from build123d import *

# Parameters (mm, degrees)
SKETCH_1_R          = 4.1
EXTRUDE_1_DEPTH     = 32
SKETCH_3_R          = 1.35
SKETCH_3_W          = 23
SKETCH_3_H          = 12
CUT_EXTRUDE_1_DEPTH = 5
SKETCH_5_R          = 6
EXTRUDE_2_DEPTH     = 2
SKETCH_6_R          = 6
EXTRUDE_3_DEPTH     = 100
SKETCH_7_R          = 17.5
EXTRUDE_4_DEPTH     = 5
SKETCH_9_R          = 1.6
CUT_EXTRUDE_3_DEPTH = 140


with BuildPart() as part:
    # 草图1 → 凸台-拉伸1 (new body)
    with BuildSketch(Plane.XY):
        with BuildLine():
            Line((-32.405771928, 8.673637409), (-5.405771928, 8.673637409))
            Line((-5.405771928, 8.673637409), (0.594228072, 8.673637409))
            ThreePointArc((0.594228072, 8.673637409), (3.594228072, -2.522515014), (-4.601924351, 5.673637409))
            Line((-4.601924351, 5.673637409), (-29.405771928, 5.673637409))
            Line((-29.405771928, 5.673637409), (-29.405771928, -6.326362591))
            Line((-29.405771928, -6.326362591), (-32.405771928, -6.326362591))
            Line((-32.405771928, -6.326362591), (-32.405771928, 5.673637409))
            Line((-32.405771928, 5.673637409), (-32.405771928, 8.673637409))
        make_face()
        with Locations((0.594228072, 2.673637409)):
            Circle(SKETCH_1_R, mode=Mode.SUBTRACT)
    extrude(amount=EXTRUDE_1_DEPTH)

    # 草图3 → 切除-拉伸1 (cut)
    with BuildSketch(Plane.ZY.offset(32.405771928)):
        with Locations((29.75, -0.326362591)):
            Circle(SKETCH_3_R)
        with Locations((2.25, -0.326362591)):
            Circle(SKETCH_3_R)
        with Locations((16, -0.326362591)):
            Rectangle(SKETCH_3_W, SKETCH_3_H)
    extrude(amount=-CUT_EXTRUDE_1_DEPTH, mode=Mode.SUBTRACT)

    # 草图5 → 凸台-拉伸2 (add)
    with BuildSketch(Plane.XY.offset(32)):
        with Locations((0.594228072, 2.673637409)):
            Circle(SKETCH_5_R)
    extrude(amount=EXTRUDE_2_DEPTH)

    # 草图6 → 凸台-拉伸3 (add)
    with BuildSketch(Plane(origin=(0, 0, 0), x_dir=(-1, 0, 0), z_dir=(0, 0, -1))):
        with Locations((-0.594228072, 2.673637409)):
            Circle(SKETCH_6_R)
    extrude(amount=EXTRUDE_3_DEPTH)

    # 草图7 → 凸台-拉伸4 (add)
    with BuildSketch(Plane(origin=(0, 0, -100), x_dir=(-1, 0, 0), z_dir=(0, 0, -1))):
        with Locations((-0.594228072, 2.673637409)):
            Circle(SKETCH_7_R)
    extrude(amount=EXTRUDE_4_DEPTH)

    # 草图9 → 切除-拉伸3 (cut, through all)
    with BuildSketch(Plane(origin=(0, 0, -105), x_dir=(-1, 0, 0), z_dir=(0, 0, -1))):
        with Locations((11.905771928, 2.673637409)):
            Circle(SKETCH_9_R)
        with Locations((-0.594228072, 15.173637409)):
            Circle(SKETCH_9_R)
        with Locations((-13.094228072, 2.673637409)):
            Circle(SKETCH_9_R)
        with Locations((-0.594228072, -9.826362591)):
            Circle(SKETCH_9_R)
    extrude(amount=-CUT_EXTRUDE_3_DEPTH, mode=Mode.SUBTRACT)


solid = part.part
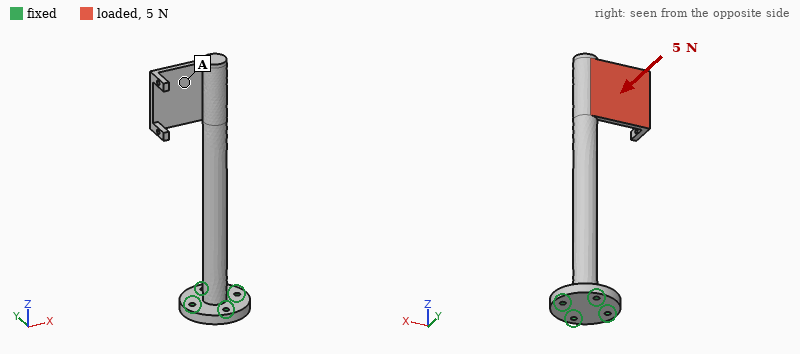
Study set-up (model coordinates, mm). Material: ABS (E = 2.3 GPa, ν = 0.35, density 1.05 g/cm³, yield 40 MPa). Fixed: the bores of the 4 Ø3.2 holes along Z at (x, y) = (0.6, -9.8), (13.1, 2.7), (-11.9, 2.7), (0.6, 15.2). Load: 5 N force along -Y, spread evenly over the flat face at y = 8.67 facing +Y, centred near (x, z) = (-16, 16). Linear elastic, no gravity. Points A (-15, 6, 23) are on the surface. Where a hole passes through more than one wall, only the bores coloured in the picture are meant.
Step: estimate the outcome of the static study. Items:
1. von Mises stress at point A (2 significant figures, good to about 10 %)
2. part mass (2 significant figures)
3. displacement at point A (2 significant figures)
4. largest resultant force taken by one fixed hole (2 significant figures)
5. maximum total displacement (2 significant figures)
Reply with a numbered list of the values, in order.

1. 0.45 MPa
2. 22 g
3. 1.5 mm
4. 26 N
5. 1.8 mm
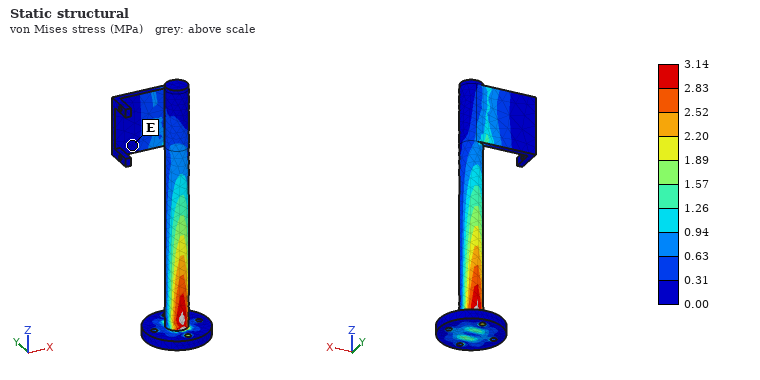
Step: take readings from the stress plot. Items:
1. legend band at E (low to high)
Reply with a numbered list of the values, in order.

1. 0.00 to 0.31 MPa
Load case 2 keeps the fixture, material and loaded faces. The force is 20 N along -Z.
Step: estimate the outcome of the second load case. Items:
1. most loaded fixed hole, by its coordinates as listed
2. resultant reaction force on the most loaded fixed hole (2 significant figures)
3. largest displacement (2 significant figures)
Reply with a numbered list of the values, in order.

1. (-11.9, 2.7)
2. 20 N
3. 1.5 mm
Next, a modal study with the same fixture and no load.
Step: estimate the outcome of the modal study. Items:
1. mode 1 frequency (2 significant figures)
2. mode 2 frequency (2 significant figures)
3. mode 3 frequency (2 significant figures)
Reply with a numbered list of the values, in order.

1. 110 Hz
2. 110 Hz
3. 470 Hz
